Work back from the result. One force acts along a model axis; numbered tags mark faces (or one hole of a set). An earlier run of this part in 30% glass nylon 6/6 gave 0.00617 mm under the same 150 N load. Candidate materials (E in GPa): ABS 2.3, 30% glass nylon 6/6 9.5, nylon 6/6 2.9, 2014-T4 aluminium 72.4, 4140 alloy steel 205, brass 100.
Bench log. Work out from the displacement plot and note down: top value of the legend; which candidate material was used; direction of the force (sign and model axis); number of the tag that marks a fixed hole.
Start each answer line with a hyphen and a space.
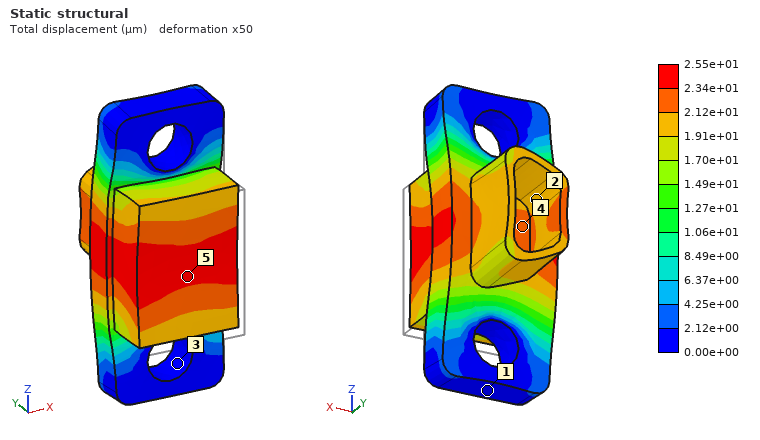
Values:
- 2.55e+01 µm
- ABS
- +Y
- 3
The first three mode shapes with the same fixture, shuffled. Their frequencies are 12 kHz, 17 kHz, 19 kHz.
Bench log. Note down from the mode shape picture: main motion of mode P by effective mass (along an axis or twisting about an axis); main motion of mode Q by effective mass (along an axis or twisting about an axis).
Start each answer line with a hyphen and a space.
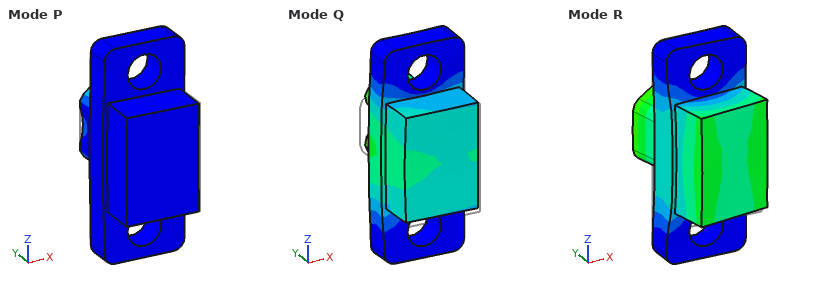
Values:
- along X
- along Y
